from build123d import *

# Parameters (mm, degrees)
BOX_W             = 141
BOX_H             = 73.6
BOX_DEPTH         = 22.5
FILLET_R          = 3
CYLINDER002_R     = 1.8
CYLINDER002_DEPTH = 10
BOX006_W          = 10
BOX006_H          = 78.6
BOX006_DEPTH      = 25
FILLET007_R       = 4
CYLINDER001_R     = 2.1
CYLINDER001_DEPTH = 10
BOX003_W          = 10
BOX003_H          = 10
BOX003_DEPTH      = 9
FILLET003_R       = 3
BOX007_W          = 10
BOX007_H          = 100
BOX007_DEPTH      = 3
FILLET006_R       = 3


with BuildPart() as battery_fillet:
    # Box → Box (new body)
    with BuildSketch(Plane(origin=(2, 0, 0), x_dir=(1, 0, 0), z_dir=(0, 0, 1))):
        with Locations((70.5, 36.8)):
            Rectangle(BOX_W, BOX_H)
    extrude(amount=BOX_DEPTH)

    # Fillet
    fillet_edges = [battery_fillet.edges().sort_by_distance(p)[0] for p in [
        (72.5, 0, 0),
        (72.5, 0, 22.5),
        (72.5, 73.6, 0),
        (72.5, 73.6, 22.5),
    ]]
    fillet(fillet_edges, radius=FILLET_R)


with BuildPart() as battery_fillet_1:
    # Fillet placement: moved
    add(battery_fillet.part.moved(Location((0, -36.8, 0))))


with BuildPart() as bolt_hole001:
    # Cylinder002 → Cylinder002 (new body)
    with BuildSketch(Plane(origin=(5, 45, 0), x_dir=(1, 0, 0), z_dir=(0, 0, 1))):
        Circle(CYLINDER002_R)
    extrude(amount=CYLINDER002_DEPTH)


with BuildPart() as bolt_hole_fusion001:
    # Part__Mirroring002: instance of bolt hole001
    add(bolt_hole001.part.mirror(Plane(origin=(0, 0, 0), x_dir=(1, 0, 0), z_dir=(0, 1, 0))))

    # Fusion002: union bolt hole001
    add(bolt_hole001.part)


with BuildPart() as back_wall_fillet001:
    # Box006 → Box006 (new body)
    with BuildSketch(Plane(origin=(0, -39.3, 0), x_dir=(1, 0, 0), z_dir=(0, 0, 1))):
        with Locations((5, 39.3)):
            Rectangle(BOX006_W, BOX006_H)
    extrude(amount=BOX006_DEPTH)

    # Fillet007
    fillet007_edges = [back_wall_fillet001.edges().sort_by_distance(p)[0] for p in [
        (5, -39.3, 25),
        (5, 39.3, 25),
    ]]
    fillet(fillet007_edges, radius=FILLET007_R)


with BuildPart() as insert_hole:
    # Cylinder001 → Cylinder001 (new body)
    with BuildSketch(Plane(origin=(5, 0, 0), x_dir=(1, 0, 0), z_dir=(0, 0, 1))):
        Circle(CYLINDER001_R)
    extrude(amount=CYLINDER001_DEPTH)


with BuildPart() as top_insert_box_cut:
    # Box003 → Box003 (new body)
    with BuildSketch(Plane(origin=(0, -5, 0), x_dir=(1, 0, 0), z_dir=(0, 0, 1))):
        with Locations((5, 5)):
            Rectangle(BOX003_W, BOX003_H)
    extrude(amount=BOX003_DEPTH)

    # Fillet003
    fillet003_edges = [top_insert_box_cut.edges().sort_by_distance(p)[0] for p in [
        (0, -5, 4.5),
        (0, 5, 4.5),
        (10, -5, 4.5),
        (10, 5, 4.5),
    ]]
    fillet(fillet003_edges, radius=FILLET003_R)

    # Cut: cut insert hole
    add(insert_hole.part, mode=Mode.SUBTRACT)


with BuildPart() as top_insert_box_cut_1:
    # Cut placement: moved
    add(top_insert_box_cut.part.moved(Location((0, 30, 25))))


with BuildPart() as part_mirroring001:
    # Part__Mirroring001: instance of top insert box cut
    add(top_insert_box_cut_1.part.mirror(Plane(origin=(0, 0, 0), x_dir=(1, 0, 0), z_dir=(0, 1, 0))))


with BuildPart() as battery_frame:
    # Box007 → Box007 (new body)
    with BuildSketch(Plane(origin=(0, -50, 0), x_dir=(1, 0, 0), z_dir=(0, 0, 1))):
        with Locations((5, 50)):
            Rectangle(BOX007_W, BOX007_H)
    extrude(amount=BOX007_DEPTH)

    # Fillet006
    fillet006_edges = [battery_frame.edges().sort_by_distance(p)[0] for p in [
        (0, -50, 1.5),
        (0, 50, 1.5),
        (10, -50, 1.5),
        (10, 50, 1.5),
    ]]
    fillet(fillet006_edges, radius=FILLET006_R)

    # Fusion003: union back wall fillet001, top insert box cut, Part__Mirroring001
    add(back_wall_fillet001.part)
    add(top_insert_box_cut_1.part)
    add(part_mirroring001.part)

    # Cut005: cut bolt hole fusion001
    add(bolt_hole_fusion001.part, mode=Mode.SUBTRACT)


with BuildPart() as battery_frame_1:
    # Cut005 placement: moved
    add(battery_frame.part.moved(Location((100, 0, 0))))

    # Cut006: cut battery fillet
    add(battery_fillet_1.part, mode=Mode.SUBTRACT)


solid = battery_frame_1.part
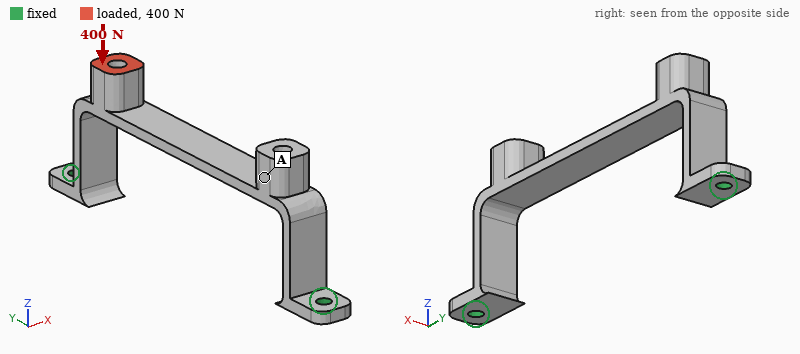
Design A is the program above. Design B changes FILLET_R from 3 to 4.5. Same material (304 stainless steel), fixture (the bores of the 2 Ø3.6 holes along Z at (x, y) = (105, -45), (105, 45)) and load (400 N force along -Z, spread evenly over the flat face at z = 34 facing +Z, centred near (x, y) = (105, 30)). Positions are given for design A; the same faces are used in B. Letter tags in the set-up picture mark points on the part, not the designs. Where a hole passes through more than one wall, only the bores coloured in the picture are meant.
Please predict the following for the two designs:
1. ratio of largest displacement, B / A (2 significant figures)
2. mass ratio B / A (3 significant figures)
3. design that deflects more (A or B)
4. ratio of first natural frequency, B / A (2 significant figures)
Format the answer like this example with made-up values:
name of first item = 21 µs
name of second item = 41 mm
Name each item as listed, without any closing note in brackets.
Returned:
ratio of largest displacement, B / A = 0.92
mass ratio B / A = 1.02
design that deflects more = A
ratio of first natural frequency, B / A = 1.0
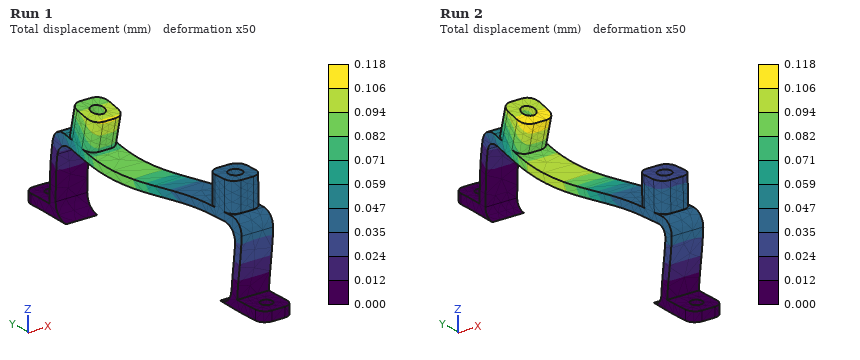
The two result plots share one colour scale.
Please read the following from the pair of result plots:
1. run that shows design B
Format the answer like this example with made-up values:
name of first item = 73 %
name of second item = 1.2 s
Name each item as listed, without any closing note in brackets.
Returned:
run that shows design B = Run 1
